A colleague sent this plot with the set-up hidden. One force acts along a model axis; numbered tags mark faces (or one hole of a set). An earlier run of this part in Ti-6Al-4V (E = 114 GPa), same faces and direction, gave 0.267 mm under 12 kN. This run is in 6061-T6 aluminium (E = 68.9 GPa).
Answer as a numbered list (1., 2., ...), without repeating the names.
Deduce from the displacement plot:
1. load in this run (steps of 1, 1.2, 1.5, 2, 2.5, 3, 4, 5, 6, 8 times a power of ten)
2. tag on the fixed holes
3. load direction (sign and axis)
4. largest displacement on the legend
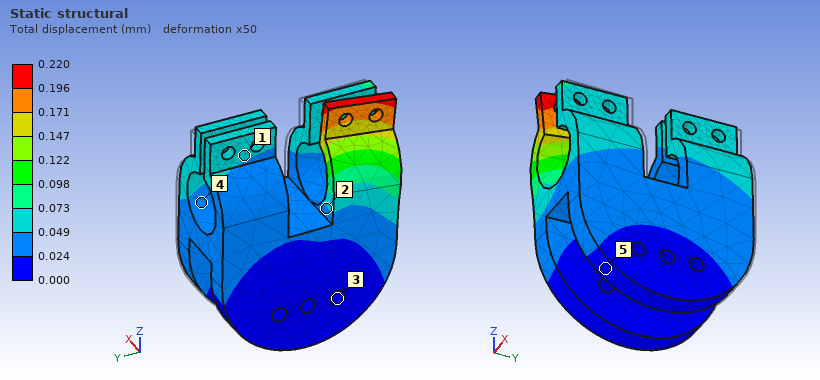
1. 6 kN
2. 3
3. -Y
4. 0.220 mm
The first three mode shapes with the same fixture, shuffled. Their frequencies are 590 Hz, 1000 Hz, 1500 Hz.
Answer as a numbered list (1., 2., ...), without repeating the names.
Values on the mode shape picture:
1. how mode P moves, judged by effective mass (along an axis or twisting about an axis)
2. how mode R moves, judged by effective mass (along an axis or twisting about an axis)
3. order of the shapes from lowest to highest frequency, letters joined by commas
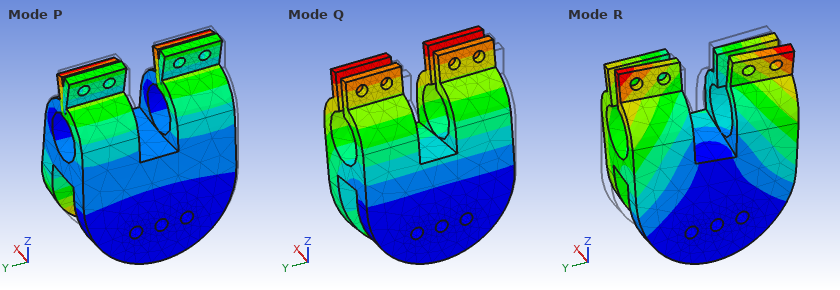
1. along X
2. along Y
3. Q, R, P
